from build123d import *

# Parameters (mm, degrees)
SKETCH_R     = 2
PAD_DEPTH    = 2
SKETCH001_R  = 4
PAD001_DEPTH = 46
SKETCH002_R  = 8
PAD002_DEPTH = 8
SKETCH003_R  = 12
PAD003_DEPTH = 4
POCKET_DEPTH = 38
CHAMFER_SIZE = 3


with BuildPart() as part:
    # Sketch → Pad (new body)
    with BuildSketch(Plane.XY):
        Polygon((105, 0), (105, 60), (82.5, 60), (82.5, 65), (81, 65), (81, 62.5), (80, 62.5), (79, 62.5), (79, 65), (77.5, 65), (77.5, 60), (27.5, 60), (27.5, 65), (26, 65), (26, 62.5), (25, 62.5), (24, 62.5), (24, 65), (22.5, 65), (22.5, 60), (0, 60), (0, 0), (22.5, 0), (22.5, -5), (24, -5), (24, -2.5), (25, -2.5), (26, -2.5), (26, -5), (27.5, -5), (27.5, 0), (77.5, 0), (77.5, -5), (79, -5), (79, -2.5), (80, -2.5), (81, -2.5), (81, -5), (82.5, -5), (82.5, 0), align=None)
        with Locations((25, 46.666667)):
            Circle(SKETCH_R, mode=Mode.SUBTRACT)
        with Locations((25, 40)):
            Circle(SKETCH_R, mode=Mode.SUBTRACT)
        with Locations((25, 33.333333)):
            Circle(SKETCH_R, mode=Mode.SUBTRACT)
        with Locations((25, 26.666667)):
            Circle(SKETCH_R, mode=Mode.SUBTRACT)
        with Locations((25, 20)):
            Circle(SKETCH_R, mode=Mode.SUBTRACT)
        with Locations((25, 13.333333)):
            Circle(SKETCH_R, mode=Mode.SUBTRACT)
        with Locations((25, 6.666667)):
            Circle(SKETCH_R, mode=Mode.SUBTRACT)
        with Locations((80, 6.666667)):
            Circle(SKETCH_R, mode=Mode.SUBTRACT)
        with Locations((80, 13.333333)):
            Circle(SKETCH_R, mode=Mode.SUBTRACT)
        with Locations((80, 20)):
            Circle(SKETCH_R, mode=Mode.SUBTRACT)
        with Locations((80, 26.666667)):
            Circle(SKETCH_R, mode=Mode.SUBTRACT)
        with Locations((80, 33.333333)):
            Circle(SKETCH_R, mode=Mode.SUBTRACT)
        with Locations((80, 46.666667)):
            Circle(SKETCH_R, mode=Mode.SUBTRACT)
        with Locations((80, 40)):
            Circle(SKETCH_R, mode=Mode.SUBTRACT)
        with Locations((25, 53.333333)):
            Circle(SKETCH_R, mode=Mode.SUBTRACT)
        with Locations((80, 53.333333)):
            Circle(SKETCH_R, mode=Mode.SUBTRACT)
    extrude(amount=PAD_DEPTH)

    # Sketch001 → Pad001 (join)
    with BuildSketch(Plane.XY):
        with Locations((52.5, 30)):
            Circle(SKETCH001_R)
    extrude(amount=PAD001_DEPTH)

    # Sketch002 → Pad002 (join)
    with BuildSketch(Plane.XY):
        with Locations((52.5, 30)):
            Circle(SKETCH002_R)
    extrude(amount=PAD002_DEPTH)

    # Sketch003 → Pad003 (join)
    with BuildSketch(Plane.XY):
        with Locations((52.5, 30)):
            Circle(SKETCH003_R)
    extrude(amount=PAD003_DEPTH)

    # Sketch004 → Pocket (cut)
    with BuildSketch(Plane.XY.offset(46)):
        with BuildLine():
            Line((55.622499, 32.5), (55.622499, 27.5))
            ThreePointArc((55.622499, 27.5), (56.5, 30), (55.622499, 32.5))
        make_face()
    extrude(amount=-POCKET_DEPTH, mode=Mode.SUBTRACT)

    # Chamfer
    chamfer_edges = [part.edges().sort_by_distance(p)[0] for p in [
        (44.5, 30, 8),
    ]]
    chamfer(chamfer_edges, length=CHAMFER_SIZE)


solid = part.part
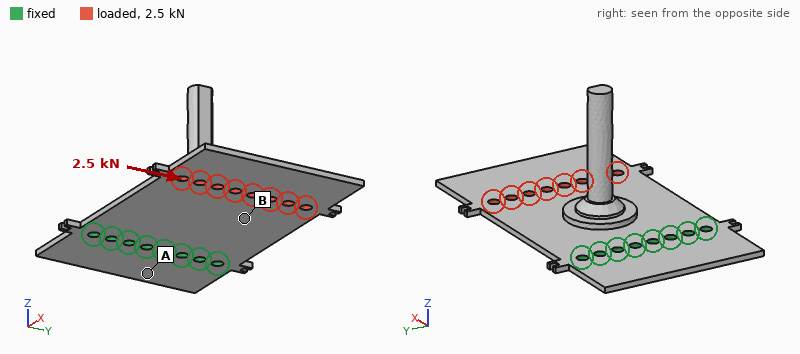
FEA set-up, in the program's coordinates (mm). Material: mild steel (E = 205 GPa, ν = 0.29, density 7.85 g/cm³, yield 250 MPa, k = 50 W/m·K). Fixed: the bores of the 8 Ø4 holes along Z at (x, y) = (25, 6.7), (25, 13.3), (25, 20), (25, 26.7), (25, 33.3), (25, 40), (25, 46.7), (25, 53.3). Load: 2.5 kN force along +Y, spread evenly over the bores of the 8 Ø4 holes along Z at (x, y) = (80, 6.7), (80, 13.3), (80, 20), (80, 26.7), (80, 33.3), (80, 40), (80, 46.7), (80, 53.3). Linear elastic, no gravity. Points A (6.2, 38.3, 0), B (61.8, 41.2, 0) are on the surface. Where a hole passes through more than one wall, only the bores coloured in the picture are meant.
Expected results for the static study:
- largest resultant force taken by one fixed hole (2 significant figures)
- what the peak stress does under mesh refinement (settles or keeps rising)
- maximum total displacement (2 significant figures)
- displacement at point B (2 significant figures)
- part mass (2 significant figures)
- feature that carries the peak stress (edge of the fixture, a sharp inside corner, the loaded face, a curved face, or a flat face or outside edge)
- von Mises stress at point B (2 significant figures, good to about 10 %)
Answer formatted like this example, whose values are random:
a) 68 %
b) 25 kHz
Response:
a) 2.1 kN
b) keeps rising
c) 60 µm
d) 23 µm
e) 120 g
f) edge of the fixture
g) 50 MPa
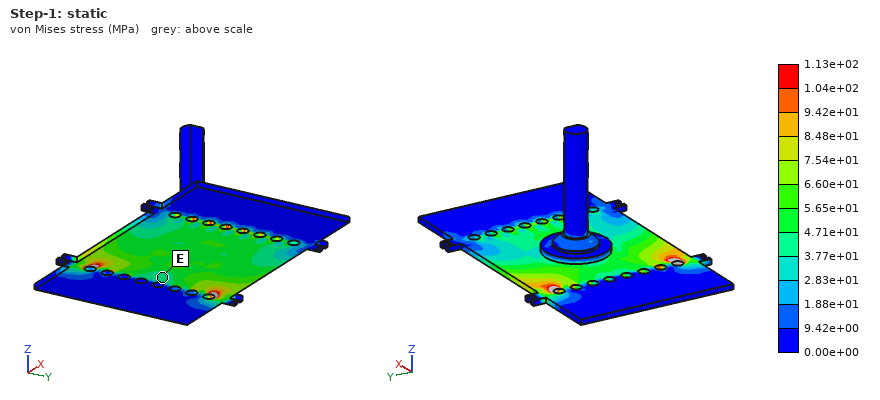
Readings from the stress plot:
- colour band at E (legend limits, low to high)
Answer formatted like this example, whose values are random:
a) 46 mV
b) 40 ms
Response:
a) 3.77e+01 to 4.71e+01 MPa
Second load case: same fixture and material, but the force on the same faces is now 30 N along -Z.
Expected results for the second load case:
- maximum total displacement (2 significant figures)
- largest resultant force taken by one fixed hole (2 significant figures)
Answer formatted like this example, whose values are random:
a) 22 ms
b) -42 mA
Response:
a) 0.23 mm
b) 15 N
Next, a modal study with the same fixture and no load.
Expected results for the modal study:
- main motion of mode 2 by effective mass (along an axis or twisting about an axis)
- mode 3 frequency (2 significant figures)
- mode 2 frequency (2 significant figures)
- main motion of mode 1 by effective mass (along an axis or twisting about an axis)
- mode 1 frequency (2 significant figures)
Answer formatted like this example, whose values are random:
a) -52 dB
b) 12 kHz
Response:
a) twisting about X
b) 1400 Hz
c) 960 Hz
d) along Z
e) 290 Hz
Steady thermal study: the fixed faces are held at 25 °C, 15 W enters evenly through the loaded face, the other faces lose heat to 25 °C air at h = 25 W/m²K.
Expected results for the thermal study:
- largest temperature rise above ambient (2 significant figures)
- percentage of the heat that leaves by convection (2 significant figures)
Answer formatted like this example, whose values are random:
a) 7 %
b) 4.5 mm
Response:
a) 63 K
b) 62 %
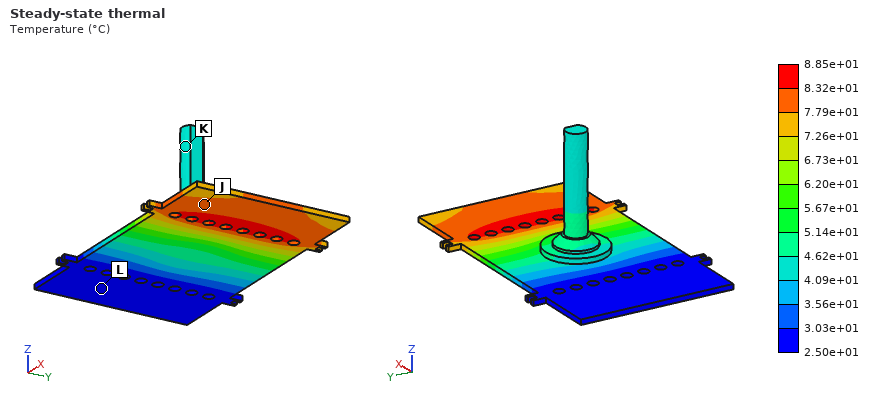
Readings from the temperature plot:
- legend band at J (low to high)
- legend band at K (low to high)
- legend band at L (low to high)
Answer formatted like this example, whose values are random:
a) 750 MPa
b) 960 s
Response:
a) 7.79e+01 to 8.32e+01 °C
b) 4.09e+01 to 4.62e+01 °C
c) 2.50e+01 to 3.03e+01 °C
